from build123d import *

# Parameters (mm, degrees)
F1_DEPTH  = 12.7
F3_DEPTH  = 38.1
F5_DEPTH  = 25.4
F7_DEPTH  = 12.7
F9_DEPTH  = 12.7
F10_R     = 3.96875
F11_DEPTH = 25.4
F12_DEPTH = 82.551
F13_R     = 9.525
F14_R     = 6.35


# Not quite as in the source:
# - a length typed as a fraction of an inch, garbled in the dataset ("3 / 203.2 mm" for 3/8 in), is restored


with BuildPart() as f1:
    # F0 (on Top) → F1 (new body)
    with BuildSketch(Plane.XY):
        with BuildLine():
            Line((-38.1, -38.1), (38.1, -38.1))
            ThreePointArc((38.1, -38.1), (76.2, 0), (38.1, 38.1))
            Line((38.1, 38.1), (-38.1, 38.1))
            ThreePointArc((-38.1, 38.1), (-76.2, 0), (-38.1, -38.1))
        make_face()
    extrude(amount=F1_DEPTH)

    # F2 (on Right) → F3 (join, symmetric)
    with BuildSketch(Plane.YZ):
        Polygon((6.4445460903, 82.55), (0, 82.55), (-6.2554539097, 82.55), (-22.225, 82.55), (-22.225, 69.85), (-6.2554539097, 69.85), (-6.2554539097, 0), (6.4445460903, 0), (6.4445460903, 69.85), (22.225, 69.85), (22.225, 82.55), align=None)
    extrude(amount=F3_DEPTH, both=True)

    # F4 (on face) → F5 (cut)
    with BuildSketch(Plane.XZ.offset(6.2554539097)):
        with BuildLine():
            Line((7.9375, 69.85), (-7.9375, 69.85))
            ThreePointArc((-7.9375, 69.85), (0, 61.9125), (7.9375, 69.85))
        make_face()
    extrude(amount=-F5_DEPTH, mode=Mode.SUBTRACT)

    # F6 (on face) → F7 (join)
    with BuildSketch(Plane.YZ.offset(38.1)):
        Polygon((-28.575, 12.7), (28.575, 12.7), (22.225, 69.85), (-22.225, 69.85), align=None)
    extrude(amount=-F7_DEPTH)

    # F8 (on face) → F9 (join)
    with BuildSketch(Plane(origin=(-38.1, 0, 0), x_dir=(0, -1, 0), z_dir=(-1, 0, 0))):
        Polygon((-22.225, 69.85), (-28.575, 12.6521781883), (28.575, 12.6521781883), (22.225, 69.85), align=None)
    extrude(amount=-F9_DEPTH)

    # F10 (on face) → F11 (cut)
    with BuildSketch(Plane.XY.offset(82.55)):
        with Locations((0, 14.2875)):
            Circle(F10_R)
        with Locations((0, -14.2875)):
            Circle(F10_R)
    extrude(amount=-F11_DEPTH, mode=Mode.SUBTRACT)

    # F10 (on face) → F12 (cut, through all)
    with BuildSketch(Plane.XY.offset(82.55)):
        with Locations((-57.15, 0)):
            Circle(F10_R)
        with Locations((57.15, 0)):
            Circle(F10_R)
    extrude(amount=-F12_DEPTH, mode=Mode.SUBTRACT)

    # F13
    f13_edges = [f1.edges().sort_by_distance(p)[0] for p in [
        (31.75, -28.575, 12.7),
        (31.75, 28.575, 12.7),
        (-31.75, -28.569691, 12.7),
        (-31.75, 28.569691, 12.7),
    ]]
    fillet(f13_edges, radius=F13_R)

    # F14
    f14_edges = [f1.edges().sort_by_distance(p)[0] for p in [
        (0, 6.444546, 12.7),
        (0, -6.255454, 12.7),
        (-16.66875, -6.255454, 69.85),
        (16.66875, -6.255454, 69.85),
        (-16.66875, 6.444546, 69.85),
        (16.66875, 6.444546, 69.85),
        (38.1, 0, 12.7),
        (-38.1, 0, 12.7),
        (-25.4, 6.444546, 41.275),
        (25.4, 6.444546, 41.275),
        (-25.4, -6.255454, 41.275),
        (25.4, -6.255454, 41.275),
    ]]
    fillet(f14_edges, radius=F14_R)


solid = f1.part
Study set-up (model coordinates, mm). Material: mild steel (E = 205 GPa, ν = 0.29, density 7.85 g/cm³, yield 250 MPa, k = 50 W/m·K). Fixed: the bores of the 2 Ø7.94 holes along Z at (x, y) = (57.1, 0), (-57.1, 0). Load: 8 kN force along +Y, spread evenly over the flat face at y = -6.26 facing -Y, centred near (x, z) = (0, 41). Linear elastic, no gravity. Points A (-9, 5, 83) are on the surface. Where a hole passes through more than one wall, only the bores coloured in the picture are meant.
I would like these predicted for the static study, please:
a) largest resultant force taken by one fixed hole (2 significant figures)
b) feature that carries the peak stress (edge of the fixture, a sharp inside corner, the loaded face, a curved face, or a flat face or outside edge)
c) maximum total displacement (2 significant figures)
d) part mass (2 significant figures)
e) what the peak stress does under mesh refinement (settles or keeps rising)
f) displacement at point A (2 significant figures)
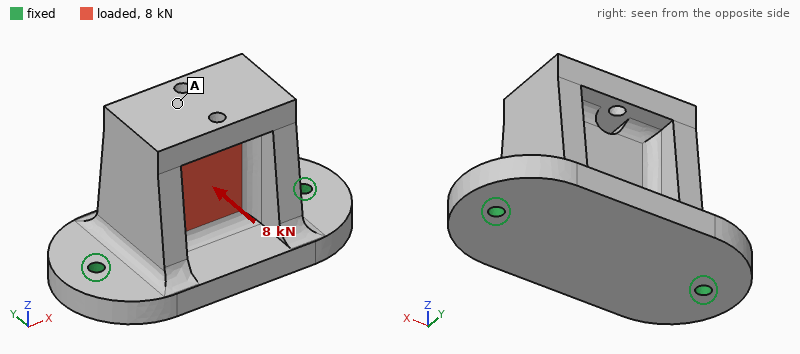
4.0 kN
edge of the fixture
90 µm
2.3 kg
keeps rising
87 µm
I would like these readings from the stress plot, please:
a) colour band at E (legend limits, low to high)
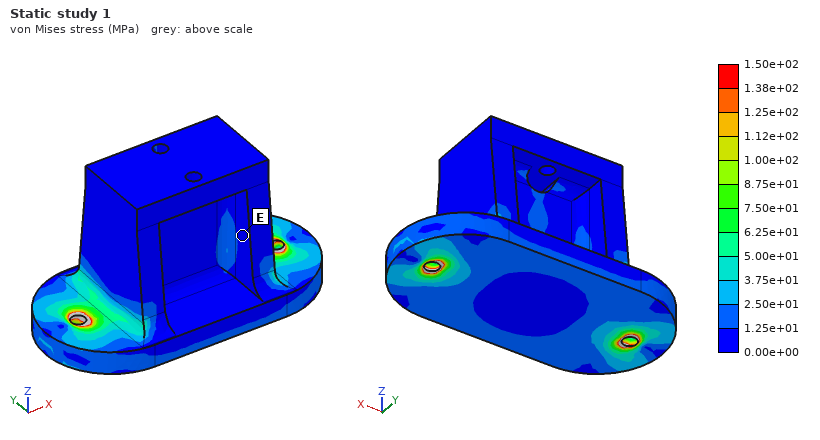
0.00e+00 to 1.25e+01 MPa
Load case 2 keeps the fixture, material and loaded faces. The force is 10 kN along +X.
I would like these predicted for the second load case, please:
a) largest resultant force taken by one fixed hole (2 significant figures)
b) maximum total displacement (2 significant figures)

6.1 kN
15 µm
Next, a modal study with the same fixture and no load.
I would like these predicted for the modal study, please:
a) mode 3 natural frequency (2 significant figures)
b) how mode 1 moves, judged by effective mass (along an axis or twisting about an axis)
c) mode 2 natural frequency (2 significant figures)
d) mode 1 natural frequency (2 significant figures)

3800 Hz
along Y
3800 Hz
1300 Hz
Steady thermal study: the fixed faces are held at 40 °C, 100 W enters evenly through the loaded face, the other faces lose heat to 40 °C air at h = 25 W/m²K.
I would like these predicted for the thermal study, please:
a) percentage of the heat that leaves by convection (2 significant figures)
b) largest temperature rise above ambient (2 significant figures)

37 %
66 K
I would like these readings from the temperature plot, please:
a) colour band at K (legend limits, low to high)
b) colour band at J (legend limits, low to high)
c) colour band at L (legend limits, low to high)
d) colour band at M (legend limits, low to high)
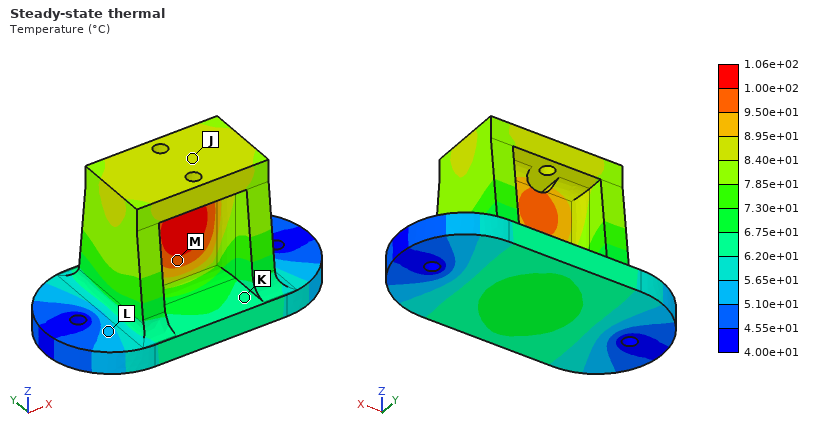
6.20e+01 to 6.75e+01 °C
8.40e+01 to 8.95e+01 °C
5.10e+01 to 5.65e+01 °C
9.50e+01 to 1.00e+02 °C
